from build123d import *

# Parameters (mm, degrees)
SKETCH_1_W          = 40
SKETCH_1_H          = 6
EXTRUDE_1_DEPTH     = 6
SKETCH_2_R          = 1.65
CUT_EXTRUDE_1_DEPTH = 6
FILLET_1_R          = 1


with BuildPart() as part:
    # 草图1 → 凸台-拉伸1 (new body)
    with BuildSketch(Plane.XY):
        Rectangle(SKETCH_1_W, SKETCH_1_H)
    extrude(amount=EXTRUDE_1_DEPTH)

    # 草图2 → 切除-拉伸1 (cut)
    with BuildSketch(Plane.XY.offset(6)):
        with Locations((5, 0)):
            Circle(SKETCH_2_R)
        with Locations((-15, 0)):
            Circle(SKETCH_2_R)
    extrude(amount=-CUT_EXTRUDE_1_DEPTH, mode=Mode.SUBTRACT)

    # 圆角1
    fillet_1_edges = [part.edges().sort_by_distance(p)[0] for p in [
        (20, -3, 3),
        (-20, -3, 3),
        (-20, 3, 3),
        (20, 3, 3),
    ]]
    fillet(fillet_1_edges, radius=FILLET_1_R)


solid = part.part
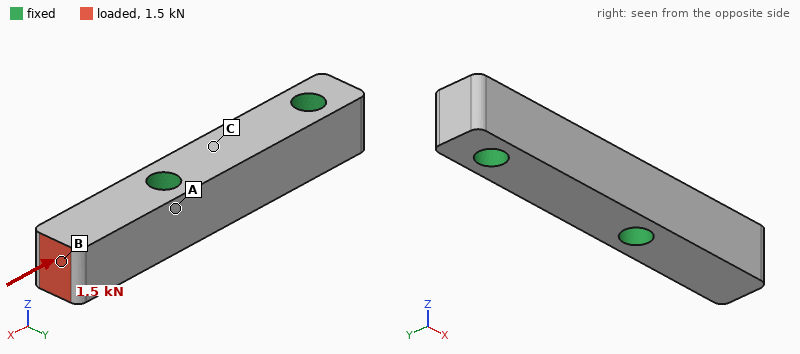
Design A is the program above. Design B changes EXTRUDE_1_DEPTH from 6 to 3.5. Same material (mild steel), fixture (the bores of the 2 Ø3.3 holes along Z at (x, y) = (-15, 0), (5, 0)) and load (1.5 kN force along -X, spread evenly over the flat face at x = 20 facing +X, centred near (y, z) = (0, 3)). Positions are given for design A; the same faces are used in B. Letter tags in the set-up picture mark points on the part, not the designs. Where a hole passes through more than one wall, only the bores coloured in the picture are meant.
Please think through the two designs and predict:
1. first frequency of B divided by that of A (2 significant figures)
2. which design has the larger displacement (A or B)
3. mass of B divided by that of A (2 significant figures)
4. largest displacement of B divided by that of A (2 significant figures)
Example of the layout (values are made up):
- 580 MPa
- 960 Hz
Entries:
- 0.71
- B
- 0.58
- 1.7
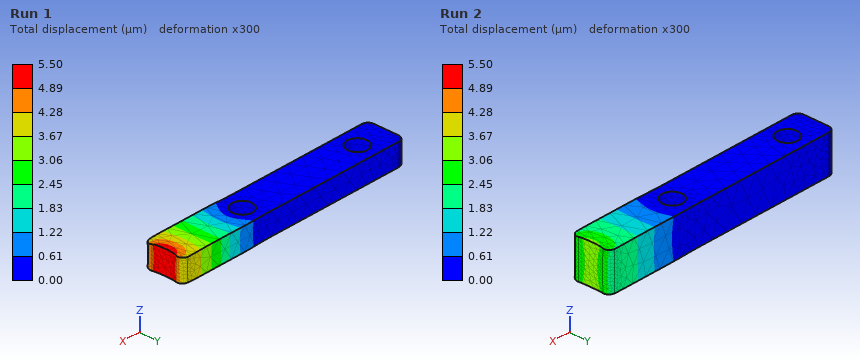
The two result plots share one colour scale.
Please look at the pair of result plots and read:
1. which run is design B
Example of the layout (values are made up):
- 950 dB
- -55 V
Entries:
- Run 1
